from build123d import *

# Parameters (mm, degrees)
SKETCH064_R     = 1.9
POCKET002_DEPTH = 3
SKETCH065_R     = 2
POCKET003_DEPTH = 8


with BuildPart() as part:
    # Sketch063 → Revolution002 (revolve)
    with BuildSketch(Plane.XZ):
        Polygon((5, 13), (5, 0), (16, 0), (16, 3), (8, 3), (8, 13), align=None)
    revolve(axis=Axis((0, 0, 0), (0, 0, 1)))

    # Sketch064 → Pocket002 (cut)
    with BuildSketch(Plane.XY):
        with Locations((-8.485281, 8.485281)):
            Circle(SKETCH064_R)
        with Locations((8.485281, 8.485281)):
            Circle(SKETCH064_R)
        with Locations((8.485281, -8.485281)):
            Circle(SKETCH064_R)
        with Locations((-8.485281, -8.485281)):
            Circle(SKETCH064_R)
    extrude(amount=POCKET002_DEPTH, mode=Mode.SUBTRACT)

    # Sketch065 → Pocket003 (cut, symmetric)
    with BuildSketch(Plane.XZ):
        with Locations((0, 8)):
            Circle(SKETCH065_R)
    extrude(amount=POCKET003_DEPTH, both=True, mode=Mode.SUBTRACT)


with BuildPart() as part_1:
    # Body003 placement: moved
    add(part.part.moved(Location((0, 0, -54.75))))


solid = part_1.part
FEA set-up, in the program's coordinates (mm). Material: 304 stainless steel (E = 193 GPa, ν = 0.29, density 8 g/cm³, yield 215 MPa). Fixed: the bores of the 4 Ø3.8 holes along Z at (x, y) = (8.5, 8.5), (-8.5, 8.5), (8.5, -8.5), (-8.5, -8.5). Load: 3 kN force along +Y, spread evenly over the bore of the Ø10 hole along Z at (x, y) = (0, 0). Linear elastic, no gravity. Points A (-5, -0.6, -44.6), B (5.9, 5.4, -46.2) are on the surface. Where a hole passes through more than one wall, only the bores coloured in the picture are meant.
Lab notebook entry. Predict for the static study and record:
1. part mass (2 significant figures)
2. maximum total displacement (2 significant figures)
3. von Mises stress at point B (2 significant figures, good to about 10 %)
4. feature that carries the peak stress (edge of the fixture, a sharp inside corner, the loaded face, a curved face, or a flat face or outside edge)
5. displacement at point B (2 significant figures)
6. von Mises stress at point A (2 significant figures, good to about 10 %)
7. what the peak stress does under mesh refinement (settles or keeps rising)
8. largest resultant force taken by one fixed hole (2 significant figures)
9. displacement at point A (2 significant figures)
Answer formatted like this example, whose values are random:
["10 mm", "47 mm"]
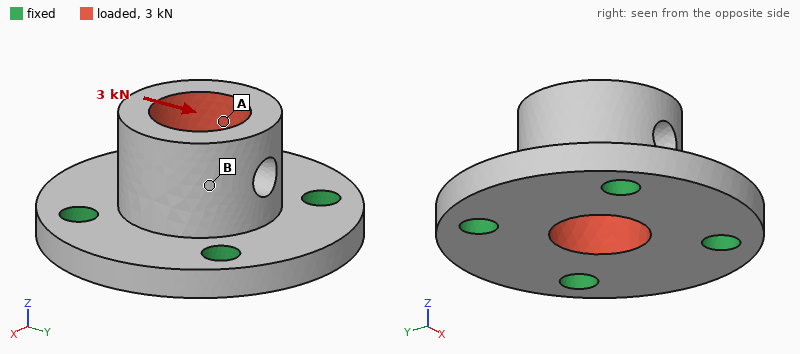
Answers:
["26 g", "7.9 µm", "15 MPa", "edge of the fixture", "4.9 µm", "35 MPa", "keeps rising", "910 N", "5.4 µm"]
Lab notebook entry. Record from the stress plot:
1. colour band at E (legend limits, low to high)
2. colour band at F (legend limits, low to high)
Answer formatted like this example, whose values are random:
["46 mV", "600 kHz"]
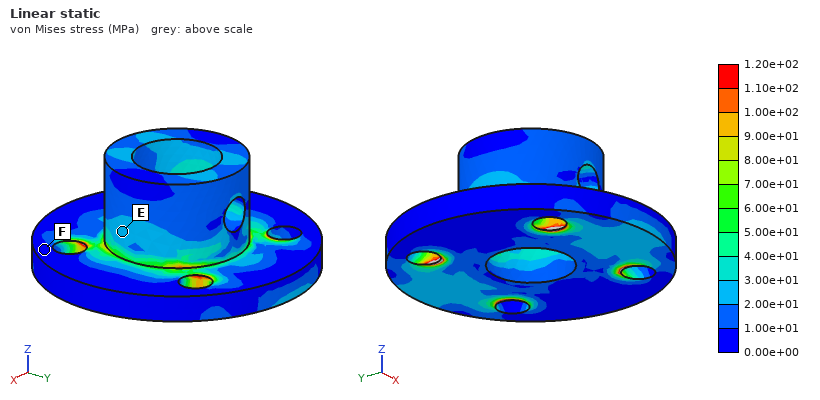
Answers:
["2.00e+01 to 3.00e+01 MPa", "0.00e+00 to 1.00e+01 MPa"]
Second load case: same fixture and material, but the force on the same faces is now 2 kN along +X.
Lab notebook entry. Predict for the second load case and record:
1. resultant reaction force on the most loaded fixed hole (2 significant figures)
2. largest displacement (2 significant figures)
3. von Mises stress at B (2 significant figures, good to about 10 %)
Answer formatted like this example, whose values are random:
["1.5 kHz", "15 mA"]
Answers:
["610 N", "6.0 µm", "15 MPa"]
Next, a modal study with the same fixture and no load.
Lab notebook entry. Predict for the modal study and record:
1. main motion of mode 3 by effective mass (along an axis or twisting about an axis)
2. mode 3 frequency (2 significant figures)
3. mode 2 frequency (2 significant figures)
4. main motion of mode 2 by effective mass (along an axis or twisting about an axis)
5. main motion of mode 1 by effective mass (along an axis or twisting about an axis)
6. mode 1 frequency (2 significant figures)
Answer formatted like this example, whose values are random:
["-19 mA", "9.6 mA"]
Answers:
["along Z", "39 kHz", "31 kHz", "along Y", "along X", "30 kHz"]
